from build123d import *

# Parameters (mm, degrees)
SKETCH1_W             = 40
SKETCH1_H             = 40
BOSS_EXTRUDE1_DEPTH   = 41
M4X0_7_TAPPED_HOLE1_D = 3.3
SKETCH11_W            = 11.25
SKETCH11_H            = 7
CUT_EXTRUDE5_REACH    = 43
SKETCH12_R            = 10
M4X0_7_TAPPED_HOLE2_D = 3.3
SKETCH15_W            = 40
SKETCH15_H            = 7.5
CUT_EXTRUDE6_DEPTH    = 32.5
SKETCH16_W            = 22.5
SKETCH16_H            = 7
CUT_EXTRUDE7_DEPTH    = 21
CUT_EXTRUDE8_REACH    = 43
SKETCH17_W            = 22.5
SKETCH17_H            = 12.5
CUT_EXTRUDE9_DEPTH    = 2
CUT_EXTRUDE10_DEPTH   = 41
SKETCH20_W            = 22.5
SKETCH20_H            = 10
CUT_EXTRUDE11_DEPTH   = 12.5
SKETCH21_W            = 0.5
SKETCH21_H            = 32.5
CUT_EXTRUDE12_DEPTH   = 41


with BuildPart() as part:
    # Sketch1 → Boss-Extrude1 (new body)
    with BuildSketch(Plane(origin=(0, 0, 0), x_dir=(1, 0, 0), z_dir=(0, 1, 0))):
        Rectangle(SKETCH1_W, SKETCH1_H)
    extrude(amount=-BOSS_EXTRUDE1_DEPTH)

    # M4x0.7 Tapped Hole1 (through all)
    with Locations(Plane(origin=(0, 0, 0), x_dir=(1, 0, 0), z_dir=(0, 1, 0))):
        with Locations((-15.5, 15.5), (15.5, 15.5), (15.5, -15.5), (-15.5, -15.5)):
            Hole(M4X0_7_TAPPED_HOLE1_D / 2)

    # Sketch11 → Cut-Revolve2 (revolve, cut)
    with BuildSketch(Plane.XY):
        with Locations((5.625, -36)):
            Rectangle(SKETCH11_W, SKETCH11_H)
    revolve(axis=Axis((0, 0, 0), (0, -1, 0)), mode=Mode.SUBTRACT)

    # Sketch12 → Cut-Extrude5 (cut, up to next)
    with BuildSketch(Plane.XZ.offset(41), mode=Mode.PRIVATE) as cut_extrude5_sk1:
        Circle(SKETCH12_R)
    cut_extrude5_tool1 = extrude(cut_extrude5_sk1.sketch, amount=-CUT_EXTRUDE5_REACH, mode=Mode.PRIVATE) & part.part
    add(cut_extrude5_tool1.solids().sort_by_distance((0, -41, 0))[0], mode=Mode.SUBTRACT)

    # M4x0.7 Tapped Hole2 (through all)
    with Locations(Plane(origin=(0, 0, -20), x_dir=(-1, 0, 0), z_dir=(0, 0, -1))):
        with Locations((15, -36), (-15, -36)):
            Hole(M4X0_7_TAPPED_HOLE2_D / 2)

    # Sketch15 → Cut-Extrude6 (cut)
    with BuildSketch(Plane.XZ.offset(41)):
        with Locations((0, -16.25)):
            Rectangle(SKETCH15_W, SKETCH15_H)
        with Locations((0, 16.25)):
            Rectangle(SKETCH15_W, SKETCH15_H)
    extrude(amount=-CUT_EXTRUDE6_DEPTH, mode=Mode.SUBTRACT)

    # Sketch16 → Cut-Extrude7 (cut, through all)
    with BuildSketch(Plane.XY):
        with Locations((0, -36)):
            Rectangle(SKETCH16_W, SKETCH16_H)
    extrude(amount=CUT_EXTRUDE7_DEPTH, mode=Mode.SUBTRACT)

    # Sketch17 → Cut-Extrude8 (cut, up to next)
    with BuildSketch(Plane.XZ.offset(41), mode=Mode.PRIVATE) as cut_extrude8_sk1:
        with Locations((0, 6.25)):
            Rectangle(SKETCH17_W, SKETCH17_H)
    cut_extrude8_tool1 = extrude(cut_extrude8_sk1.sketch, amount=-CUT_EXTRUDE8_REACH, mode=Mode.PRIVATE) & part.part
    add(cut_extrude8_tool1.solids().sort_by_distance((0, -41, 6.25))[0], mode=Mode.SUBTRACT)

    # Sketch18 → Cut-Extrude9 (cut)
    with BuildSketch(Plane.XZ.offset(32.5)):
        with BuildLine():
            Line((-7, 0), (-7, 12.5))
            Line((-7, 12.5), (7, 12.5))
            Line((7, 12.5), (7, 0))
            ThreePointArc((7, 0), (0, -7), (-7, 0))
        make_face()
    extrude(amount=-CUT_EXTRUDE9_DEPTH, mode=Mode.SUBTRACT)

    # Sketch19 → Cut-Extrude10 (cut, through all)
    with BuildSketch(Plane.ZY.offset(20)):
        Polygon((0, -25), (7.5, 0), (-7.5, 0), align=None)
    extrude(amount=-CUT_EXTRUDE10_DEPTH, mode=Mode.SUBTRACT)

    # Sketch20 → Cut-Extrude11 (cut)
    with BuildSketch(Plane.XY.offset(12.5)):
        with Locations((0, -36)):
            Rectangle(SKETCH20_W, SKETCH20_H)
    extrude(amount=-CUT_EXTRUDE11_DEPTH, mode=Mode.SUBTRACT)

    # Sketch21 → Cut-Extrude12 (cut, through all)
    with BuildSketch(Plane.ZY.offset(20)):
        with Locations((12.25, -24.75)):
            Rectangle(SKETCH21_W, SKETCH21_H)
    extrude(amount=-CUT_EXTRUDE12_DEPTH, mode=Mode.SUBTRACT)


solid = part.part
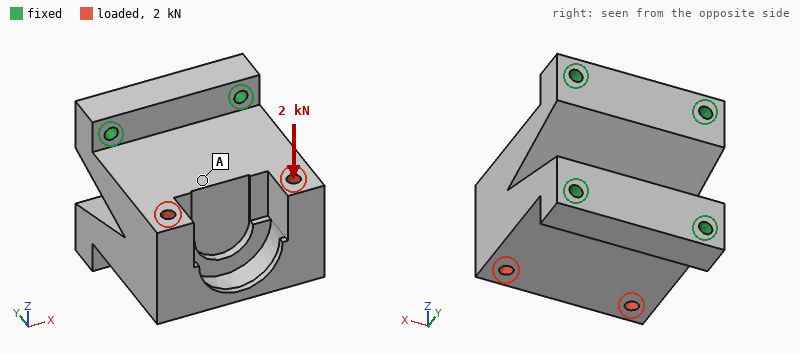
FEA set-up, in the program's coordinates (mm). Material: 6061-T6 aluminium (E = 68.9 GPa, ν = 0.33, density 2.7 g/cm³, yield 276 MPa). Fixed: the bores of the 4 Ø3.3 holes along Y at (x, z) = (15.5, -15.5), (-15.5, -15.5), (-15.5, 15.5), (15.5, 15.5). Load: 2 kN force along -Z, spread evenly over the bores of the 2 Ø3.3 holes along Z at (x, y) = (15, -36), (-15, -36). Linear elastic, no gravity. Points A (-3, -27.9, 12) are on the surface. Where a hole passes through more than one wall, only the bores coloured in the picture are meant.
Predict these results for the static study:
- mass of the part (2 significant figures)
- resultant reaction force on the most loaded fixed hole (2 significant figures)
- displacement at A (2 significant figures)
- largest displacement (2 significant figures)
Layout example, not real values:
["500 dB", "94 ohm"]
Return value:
["88 g", "1.3 kN", "13 µm", "22 µm"]
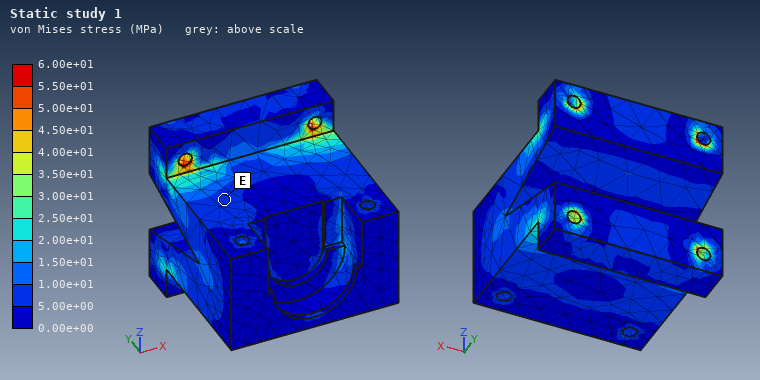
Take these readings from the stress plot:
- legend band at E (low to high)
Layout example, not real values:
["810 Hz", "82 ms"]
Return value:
["5.00e+00 to 1.00e+01 MPa"]
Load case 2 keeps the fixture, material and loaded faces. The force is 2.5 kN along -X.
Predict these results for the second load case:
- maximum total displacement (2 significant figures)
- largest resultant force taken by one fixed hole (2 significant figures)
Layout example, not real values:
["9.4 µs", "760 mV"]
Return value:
["27 µm", "1.5 kN"]
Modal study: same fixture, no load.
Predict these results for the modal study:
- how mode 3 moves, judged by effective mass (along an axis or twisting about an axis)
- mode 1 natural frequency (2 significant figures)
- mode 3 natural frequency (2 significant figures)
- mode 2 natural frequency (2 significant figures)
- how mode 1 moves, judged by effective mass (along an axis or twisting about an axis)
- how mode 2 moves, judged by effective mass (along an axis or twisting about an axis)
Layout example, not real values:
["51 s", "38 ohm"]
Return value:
["twisting about Y", "10000 Hz", "15 kHz", "10 kHz", "along Z", "along X"]
